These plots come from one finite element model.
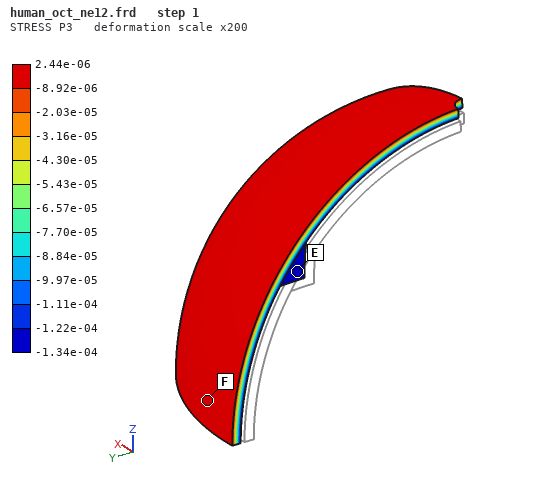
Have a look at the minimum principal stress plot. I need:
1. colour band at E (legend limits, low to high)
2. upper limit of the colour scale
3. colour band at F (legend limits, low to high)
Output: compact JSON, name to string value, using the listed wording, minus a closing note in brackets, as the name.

{"colour band at E": "-1.34e-04 to -1.22e-04", "upper limit of the colour scale": "2.44e-06", "colour band at F": "-8.92e-06 to 2.44e-06"}
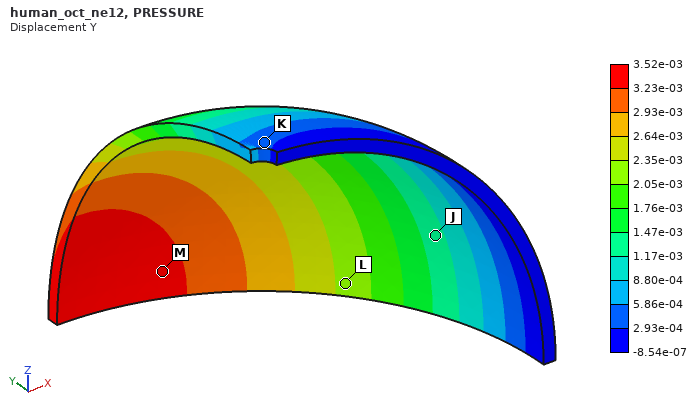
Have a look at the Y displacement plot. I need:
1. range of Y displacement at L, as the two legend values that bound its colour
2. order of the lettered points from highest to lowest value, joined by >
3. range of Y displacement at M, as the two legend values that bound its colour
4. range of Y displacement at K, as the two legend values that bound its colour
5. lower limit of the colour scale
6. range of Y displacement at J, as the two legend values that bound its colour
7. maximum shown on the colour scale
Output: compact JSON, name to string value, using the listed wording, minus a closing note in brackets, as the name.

{"range of Y displacement at L, as the two legend values that bound its colour": "2.05e-03 to 2.35e-03", "order of the lettered points from highest to lowest value, joined by >": "M > L > J > K", "range of Y displacement at M, as the two legend values that bound its colour": "3.23e-03 to 3.52e-03", "range of Y displacement at K, as the two legend values that bound its colour": "2.93e-04 to 5.86e-04", "lower limit of the colour scale": "-8.54e-07", "range of Y displacement at J, as the two legend values that bound its colour": "1.17e-03 to 1.47e-03", "maximum shown on the colour scale": "3.52e-03"}
